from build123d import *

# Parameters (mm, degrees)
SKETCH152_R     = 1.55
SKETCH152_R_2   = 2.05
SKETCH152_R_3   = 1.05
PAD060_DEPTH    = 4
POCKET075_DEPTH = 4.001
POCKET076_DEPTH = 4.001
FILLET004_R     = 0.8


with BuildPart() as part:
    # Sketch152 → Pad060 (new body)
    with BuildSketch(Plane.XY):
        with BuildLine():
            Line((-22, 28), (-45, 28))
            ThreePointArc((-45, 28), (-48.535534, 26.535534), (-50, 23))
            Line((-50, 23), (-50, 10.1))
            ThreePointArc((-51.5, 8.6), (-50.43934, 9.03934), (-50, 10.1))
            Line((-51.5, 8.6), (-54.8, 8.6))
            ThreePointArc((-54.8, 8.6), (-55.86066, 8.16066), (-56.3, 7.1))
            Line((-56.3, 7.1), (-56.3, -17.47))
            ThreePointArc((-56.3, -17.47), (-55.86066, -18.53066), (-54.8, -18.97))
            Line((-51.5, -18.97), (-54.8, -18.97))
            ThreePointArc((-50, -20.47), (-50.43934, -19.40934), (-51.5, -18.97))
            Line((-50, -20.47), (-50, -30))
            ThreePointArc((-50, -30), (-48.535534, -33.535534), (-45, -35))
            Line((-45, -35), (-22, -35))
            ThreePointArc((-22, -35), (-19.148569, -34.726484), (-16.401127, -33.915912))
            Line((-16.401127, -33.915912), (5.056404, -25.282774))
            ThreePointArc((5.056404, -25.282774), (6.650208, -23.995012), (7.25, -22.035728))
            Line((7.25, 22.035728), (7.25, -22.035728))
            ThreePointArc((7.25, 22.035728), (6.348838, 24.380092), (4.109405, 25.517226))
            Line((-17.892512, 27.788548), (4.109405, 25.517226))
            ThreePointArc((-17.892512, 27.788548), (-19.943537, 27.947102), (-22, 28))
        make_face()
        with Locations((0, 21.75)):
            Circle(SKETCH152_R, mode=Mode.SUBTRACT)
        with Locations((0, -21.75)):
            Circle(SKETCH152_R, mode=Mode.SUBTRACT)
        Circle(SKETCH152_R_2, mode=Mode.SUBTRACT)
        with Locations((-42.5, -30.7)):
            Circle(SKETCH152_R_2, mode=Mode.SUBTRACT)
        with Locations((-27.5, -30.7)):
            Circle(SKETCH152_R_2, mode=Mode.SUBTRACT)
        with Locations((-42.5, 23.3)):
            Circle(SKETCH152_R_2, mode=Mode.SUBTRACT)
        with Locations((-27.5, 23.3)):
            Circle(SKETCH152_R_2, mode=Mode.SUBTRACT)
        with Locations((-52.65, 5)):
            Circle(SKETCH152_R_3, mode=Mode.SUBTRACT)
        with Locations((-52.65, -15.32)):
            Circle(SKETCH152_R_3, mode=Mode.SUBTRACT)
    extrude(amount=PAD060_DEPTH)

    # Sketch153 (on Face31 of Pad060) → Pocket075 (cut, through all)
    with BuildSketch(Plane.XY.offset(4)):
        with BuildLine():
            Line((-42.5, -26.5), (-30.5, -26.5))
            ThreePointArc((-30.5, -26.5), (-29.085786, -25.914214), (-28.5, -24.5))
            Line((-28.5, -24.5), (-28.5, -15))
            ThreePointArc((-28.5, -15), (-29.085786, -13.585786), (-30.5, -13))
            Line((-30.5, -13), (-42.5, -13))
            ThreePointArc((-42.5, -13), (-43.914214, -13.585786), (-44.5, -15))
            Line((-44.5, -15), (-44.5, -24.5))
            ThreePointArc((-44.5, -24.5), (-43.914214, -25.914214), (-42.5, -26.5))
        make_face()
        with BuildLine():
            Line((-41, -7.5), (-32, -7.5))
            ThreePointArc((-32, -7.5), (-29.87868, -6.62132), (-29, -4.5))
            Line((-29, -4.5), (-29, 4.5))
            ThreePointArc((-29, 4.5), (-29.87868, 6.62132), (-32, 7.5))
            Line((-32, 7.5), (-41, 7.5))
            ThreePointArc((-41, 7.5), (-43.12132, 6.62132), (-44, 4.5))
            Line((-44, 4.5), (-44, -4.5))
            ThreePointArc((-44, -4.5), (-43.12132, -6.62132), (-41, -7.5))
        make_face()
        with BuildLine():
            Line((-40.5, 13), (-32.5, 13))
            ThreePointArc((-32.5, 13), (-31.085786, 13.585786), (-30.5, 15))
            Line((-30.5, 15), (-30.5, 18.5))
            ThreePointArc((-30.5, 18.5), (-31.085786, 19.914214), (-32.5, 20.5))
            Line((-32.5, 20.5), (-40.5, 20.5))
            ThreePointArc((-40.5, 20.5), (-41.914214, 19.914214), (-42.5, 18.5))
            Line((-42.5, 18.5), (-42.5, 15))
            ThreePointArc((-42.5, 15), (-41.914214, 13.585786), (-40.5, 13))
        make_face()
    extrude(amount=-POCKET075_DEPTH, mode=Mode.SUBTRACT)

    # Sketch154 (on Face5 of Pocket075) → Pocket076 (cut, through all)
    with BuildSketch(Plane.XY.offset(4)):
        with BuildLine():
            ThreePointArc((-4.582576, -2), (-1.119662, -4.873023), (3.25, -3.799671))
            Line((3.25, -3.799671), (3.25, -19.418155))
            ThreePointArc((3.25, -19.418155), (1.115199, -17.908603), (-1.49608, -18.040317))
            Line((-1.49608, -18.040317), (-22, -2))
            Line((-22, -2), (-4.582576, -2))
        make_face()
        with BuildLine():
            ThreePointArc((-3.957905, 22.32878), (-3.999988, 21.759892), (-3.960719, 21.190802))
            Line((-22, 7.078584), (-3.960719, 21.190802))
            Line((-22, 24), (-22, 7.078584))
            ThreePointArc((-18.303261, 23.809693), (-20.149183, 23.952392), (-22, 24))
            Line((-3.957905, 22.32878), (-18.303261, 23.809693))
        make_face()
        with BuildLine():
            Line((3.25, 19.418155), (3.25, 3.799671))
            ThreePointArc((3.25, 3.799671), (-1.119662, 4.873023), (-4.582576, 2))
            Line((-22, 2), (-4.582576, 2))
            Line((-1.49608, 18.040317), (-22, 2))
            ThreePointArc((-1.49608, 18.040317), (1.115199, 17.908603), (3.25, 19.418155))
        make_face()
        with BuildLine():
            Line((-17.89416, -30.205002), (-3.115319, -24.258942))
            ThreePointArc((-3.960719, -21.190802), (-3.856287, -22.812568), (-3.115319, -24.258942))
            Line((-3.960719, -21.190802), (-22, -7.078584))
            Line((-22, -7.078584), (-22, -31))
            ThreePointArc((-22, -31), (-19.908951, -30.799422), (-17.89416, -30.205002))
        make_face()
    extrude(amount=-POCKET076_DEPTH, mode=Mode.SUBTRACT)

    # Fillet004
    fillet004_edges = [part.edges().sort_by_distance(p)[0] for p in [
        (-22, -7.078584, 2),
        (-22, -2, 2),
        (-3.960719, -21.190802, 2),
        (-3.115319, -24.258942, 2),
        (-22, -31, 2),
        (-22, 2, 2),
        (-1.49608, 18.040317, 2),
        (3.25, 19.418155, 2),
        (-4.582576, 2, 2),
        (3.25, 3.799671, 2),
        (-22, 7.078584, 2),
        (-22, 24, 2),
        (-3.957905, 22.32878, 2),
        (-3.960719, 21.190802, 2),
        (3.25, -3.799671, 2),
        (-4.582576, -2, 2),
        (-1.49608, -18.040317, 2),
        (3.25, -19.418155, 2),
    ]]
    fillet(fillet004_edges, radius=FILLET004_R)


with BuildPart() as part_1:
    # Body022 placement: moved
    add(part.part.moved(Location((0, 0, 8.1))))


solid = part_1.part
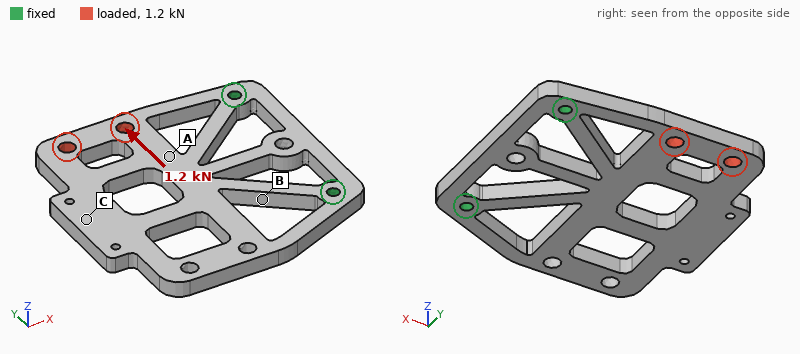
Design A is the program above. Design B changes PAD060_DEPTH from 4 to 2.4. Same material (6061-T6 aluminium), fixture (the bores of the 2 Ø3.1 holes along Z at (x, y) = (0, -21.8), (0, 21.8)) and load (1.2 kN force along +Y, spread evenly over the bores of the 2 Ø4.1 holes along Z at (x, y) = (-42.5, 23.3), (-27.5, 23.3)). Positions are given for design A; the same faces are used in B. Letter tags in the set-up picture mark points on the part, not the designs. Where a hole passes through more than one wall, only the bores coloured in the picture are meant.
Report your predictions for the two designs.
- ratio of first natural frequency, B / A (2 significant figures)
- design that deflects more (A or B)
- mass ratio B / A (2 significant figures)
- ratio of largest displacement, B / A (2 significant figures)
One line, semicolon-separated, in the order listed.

0.62; B; 0.60; 1.7
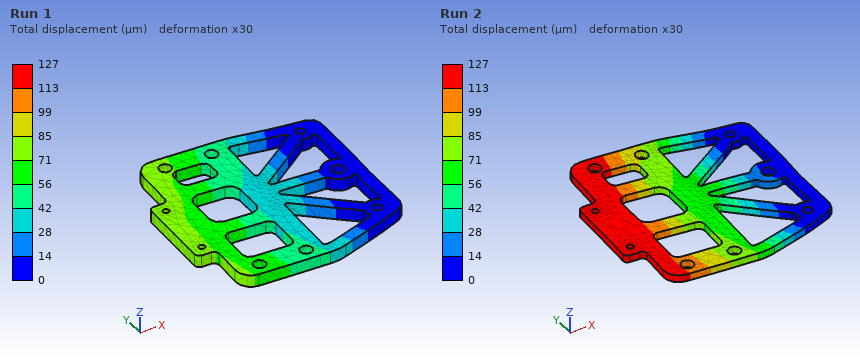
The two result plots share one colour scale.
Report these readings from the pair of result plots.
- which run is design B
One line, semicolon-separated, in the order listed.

Run 2
